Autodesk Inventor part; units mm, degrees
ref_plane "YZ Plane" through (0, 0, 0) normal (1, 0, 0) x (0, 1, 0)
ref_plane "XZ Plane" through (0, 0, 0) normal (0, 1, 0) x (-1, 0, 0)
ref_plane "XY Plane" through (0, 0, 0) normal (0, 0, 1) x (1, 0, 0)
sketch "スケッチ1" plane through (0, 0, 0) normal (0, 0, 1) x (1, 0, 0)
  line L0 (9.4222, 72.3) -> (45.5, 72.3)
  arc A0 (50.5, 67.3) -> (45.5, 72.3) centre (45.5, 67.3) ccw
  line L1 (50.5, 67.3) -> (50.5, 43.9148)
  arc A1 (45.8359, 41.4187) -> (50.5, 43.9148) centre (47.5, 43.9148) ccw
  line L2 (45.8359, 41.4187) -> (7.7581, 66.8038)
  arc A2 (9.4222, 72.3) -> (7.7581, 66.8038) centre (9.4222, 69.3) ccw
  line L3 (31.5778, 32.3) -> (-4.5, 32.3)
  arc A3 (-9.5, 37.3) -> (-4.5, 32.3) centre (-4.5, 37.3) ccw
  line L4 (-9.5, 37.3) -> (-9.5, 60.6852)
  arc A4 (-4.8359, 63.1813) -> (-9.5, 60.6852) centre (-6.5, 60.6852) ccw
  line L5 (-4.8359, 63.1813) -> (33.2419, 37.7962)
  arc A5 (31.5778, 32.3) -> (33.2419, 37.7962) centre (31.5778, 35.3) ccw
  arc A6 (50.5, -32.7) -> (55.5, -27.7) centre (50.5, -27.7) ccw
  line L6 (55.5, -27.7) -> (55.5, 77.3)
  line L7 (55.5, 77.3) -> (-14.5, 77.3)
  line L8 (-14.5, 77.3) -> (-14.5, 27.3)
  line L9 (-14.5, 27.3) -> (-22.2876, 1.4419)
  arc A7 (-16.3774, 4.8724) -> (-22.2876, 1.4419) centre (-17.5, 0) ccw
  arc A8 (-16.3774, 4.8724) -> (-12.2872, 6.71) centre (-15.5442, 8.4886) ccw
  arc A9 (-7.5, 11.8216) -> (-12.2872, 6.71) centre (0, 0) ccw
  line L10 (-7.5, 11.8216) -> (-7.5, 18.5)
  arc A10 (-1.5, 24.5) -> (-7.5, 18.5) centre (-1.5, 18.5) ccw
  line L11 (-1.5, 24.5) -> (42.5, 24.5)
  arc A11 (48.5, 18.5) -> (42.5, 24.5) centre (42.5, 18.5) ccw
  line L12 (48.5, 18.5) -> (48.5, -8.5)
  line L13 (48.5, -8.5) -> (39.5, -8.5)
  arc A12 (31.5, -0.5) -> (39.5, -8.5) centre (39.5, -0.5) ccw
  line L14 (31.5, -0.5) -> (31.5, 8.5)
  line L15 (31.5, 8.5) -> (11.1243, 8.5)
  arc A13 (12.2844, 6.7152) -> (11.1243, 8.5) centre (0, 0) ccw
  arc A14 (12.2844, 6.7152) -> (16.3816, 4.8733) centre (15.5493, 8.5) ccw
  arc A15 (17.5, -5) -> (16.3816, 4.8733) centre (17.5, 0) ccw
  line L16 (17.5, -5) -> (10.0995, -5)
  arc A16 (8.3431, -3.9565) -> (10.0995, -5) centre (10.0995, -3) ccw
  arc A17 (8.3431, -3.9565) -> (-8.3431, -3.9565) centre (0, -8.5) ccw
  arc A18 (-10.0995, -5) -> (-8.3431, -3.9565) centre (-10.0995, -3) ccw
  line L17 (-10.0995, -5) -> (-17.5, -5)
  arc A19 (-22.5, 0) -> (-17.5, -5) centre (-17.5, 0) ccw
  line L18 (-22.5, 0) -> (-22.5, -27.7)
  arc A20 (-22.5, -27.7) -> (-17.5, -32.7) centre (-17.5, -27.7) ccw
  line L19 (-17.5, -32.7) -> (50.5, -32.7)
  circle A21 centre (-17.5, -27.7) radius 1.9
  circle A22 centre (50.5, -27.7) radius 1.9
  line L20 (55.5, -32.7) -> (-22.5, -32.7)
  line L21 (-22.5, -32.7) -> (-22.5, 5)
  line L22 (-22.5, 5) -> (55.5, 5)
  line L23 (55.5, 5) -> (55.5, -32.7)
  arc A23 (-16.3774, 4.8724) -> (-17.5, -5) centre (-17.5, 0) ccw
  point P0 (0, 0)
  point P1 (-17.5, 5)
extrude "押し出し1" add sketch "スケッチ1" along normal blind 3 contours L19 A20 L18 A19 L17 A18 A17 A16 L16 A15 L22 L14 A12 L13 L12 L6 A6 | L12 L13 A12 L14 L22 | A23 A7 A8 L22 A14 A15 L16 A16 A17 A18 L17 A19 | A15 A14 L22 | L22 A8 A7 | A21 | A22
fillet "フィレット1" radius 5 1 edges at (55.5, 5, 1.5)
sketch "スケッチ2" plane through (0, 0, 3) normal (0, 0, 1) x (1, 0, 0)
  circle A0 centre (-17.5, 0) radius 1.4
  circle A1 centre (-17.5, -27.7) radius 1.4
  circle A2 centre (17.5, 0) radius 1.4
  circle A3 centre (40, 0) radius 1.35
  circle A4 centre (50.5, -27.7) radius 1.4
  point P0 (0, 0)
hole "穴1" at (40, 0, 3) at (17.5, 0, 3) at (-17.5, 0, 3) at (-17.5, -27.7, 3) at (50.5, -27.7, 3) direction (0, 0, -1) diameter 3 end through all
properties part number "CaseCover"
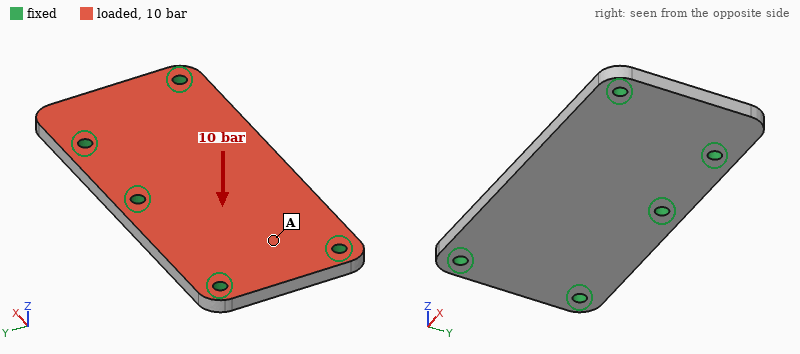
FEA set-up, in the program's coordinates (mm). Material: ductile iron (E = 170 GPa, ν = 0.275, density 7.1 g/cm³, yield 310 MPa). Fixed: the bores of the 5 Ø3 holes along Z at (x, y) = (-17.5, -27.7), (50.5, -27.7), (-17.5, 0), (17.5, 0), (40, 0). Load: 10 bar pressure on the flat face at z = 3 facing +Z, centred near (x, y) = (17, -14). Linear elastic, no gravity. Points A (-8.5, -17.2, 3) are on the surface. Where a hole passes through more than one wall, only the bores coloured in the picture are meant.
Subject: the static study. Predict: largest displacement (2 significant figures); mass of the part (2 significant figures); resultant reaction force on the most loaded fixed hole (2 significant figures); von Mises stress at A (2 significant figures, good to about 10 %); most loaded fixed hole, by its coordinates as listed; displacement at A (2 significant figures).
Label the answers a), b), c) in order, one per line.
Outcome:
a) 0.11 mm
b) 61 g
c) 860 N
d) 52 MPa
e) (17.5, 0)
f) 0.023 mm
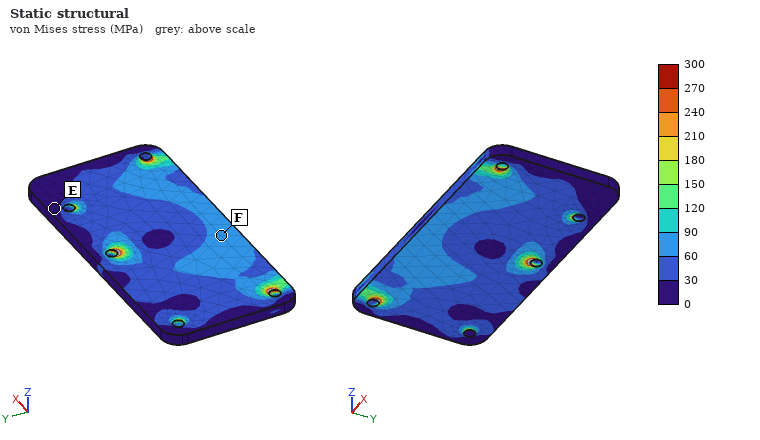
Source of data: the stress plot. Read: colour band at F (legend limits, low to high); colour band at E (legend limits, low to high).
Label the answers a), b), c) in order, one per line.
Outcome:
a) 60 to 90 MPa
b) 0 to 30 MPa
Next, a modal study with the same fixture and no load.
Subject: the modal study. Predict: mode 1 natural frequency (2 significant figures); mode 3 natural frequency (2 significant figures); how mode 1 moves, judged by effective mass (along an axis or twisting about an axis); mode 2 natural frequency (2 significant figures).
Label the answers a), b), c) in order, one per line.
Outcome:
a) 4500 Hz
b) 11 kHz
c) along Z
d) 9200 Hz
